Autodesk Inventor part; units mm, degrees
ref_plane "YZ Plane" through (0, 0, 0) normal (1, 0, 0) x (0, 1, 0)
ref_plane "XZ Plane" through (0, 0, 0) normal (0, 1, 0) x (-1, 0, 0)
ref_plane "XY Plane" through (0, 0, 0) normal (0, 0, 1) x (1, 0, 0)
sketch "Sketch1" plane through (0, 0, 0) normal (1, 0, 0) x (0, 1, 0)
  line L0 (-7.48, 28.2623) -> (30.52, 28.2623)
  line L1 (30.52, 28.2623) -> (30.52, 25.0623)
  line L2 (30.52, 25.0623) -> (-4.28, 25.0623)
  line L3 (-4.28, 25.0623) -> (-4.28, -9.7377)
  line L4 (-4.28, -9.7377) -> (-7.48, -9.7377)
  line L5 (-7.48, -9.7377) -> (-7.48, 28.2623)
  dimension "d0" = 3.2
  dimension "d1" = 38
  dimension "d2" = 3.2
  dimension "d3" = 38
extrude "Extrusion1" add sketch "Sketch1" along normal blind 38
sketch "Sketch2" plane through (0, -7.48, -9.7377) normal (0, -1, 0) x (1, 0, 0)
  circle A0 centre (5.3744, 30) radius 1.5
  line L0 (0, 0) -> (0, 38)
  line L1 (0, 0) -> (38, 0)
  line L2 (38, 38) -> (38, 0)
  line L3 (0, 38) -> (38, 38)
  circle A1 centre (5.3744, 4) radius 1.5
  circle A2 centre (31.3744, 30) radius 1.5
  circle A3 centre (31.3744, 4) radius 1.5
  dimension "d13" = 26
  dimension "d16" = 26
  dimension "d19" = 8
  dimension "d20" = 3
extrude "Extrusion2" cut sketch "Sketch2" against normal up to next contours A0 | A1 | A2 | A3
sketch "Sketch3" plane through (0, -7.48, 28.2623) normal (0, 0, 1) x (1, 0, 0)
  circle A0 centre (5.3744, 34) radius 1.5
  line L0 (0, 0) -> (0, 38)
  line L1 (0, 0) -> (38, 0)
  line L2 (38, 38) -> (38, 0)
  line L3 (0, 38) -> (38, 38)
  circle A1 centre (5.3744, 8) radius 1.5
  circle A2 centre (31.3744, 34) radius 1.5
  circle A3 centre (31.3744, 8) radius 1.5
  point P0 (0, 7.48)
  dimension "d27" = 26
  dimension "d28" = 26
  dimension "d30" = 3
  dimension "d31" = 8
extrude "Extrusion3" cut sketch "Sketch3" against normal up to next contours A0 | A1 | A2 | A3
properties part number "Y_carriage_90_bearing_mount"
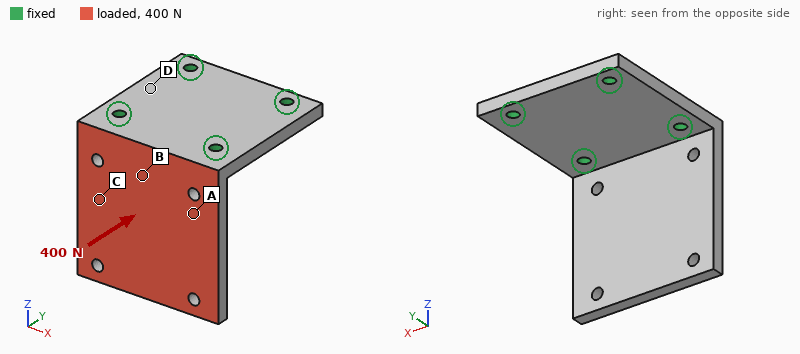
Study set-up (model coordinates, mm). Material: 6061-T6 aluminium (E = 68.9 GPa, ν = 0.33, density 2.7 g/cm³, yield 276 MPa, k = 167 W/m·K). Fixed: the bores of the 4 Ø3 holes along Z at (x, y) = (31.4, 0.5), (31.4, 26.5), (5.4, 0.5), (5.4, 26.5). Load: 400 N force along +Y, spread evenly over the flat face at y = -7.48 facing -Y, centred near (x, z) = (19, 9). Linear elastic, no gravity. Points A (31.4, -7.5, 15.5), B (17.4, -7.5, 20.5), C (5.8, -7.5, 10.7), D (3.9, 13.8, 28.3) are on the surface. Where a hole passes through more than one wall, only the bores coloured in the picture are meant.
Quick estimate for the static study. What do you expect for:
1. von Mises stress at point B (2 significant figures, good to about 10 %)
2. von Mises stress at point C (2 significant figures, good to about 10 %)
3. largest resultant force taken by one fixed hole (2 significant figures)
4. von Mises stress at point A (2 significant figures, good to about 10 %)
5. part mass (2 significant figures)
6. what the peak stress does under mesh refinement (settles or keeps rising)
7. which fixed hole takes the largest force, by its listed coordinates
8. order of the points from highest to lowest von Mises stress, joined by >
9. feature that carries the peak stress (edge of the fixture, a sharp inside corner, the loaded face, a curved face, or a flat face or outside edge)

69 MPa
33 MPa
170 N
42 MPa
23 g
keeps rising
(31.4, 0.5)
B > A > C > D
edge of the fixture
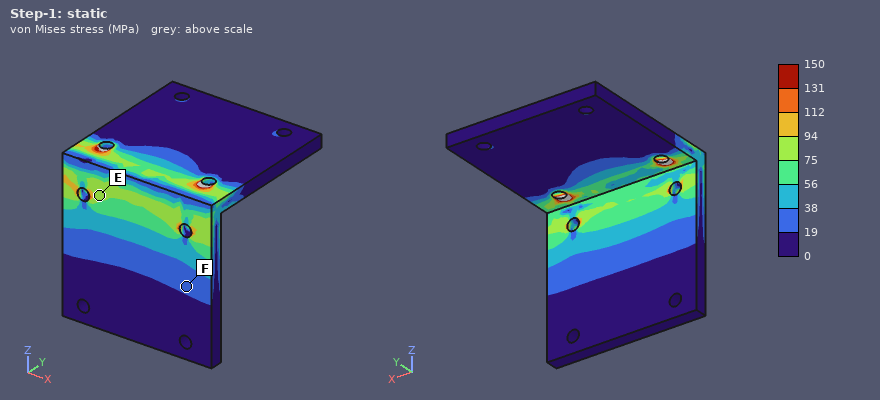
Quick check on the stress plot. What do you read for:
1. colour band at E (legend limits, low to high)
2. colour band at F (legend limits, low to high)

75 to 94 MPa
19 to 38 MPa
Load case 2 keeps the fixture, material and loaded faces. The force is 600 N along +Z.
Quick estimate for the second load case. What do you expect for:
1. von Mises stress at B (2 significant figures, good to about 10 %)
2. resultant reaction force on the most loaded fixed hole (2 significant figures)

14 MPa
340 N
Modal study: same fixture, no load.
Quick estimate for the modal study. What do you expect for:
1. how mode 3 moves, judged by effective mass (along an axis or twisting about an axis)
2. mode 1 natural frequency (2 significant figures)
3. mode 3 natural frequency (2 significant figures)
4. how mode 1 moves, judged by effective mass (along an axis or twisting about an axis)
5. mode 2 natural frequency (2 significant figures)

along X
1600 Hz
6900 Hz
along Y
4100 Hz
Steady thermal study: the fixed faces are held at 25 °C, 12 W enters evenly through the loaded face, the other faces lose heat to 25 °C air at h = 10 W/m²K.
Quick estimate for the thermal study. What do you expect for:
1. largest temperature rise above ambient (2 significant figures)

15 K
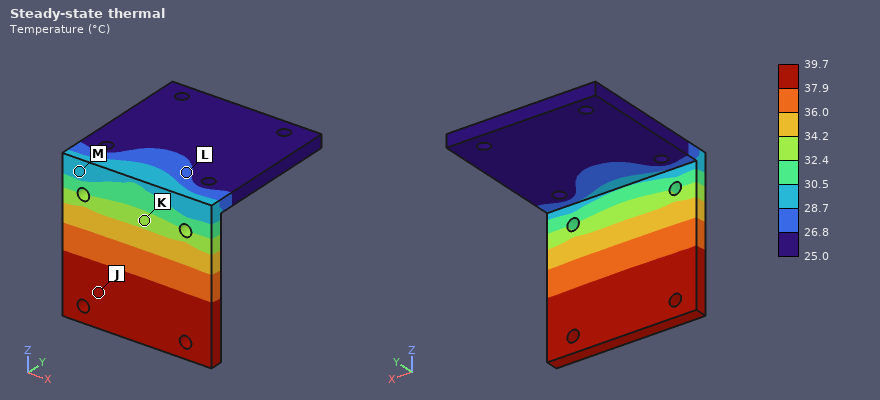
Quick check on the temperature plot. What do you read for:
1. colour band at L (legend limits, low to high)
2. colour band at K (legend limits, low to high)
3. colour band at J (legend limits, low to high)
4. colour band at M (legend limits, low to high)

26.8 to 28.7 °C
32.4 to 34.2 °C
37.9 to 39.7 °C
28.7 to 30.5 °C
